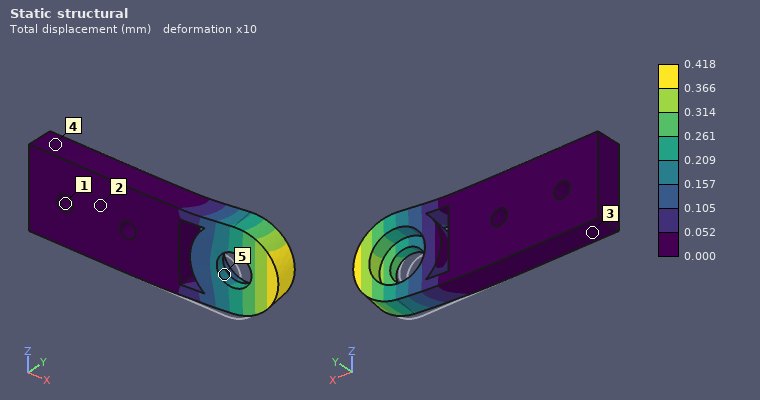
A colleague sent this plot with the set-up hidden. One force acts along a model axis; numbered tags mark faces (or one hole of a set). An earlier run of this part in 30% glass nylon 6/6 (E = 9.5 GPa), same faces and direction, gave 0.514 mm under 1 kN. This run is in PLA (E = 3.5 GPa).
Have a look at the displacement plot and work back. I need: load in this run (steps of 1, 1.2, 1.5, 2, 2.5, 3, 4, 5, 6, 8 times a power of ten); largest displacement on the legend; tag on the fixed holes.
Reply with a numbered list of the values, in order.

1. 300 N
2. 0.418 mm
3. 1
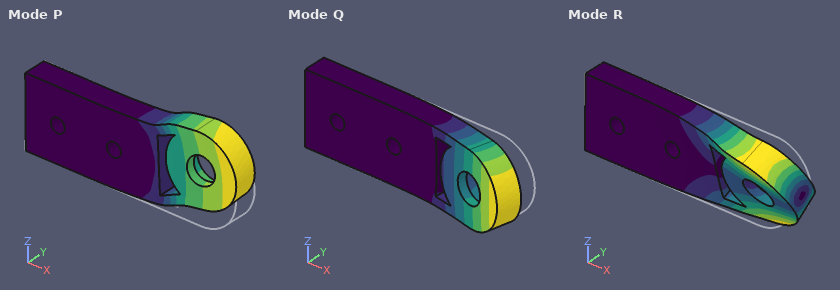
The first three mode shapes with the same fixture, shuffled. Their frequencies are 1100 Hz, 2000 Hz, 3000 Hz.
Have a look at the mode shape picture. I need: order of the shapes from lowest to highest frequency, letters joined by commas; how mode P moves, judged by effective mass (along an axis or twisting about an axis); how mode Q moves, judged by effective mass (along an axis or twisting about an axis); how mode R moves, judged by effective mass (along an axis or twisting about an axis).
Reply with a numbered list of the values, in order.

1. Q, P, R
2. along Z
3. along Y
4. twisting about X
